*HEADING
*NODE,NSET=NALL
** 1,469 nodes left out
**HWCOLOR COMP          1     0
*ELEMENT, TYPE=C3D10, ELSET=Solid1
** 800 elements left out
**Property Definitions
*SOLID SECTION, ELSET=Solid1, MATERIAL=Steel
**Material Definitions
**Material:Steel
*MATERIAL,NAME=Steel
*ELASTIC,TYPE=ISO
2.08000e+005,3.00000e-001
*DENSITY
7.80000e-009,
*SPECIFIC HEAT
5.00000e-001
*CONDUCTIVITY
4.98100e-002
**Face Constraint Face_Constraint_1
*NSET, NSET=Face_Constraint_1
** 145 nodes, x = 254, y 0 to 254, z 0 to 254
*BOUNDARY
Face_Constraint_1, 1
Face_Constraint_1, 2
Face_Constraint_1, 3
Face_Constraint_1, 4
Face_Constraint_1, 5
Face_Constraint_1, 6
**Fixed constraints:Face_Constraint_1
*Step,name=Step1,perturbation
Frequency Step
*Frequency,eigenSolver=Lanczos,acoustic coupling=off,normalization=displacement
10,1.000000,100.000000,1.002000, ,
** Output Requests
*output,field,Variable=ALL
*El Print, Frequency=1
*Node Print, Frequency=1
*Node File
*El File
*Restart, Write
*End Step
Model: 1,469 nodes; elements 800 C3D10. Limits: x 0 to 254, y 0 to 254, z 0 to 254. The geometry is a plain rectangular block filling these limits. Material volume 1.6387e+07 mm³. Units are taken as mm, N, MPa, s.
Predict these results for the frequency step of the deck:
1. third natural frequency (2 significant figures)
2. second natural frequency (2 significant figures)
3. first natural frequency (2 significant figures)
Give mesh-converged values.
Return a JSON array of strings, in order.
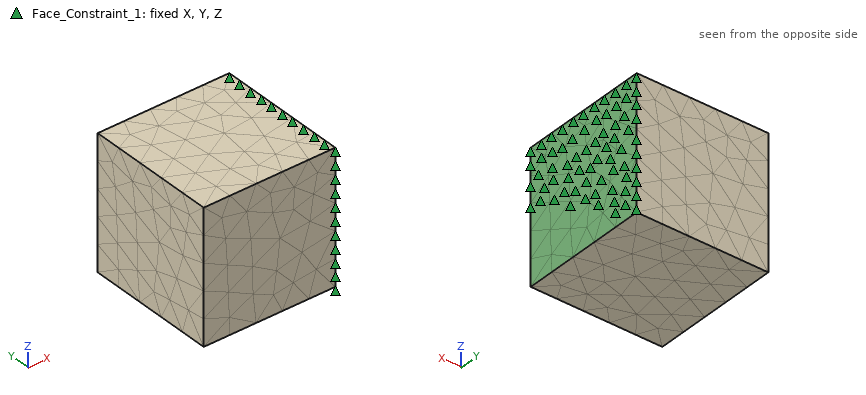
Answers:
["2900 Hz", "2200 Hz", "2200 Hz"]
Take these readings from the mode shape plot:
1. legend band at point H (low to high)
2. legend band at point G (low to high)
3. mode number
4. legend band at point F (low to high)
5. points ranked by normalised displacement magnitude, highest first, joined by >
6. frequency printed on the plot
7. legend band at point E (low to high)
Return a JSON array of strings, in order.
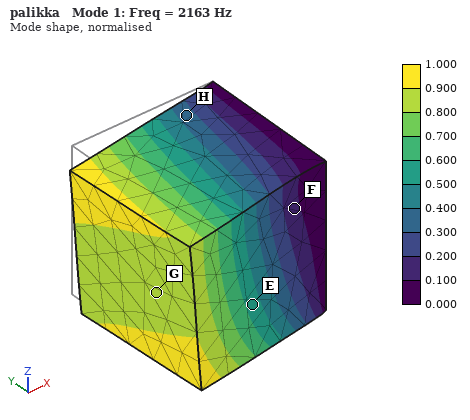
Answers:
["0.300 to 0.400", "0.800 to 0.900", "1", "0.100 to 0.200", "G > E > H > F", "2163 Hz", "0.500 to 0.600"]
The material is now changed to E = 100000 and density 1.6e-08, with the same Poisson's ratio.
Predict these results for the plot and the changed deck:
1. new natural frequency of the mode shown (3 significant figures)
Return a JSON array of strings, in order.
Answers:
["1050 Hz"]
